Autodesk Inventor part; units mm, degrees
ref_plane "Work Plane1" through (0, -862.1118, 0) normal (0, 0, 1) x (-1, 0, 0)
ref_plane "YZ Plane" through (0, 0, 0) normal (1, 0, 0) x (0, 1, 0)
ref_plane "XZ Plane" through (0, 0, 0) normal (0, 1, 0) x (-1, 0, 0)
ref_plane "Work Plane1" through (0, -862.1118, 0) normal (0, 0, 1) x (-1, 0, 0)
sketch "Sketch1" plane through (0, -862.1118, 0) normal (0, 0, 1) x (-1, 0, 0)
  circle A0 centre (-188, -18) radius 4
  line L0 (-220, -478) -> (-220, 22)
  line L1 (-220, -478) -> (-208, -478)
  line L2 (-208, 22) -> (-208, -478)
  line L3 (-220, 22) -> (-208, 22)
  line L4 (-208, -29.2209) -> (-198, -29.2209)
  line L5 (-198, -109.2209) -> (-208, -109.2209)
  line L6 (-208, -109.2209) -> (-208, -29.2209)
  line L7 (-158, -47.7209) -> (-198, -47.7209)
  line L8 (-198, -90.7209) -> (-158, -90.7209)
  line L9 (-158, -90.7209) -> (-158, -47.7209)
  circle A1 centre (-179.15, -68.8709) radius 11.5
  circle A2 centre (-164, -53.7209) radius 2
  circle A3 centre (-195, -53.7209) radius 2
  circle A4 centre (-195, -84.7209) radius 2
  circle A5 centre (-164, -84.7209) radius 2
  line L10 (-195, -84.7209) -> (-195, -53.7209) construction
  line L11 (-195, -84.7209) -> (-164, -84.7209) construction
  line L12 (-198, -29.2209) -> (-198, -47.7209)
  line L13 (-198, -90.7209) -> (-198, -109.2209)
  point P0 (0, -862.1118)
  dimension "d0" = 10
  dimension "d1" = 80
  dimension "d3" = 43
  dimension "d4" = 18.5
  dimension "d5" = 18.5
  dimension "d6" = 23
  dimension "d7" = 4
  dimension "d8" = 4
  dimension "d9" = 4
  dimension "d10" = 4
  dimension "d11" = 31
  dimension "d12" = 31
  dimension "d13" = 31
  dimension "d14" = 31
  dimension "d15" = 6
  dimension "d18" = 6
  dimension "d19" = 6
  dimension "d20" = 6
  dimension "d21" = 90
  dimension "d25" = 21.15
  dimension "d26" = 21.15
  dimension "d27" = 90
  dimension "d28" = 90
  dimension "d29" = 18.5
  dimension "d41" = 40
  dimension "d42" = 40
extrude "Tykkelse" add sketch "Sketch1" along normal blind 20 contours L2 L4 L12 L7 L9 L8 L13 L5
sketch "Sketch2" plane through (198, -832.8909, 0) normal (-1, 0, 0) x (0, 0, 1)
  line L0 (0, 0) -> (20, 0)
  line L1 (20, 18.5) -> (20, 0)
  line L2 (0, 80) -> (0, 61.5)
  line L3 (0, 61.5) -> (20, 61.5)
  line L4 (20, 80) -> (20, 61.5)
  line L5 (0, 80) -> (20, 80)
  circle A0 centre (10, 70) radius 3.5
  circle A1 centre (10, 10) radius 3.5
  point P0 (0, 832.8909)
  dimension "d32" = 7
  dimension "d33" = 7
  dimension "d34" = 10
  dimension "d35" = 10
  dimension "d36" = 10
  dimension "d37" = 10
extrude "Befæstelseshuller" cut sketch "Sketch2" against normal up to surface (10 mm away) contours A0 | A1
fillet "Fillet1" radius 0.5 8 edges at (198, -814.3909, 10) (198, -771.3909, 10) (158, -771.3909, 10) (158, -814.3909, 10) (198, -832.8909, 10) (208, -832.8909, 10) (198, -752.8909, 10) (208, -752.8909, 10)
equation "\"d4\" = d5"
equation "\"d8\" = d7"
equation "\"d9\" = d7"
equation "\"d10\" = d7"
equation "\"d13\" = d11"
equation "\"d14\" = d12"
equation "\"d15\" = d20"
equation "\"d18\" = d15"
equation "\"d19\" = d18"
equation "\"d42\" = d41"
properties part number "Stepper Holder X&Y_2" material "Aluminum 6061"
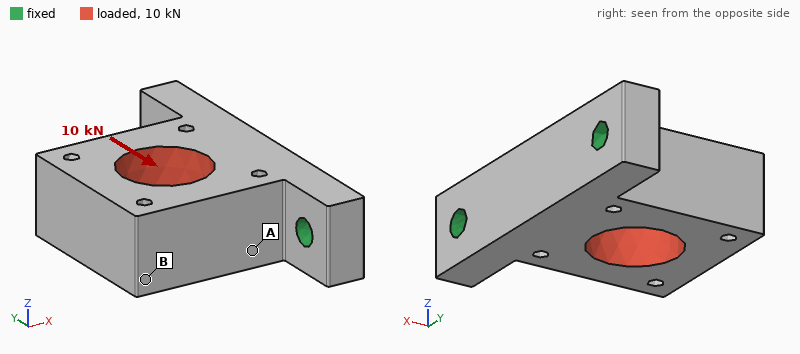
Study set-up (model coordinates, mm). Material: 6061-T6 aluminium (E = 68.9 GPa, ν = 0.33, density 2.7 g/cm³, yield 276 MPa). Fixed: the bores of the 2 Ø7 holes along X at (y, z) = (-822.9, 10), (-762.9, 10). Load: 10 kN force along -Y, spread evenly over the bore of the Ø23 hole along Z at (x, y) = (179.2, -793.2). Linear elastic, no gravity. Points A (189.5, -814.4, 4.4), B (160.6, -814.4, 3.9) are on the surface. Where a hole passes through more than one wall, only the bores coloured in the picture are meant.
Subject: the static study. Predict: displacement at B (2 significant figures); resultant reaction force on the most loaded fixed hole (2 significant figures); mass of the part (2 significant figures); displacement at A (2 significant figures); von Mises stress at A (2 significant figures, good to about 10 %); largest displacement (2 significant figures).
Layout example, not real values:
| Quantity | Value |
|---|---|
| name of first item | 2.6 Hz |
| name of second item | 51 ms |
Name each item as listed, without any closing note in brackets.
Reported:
| Quantity | Value |
|---|---|
| displacement at B | 78 µm |
| resultant reaction force on the most loaded fixed hole | 6.9 kN |
| mass of the part | 110 g |
| displacement at A | 29 µm |
| von Mises stress at A | 46 MPa |
| largest displacement | 81 µm |
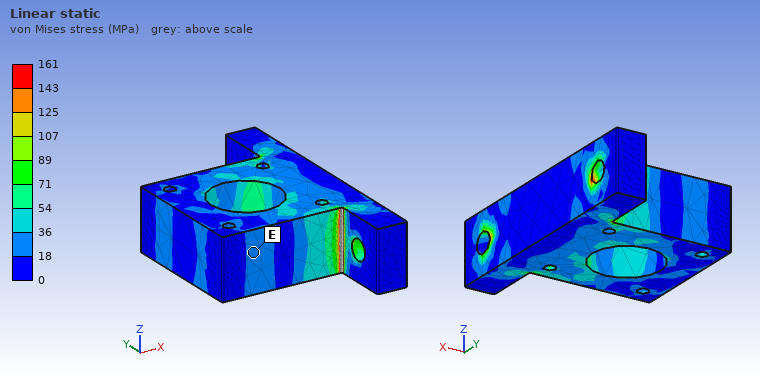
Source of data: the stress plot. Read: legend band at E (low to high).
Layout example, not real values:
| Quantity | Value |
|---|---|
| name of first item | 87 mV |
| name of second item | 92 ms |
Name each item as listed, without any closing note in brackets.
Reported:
| Quantity | Value |
|---|---|
| legend band at E | 18 to 36 MPa |
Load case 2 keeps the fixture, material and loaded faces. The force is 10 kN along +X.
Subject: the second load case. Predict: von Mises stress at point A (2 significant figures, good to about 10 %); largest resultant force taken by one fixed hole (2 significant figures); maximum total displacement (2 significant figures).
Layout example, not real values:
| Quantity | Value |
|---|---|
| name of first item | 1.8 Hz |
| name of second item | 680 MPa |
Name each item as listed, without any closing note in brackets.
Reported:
| Quantity | Value |
|---|---|
| von Mises stress at point A | 30 MPa |
| largest resultant force taken by one fixed hole | 5.4 kN |
| maximum total displacement | 29 µm |
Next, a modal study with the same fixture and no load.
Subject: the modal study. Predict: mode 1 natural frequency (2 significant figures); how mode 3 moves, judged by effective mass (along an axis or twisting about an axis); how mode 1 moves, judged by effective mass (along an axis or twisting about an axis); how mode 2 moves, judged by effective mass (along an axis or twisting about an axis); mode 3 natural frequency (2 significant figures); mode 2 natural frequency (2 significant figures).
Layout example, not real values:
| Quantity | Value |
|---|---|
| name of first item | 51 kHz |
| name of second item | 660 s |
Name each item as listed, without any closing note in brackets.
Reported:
| Quantity | Value |
|---|---|
| mode 1 natural frequency | 3000 Hz |
| how mode 3 moves, judged by effective mass | twisting about X |
| how mode 1 moves, judged by effective mass | along Z |
| how mode 2 moves, judged by effective mass | along Y |
| mode 3 natural frequency | 9500 Hz |
| mode 2 natural frequency | 7300 Hz |
